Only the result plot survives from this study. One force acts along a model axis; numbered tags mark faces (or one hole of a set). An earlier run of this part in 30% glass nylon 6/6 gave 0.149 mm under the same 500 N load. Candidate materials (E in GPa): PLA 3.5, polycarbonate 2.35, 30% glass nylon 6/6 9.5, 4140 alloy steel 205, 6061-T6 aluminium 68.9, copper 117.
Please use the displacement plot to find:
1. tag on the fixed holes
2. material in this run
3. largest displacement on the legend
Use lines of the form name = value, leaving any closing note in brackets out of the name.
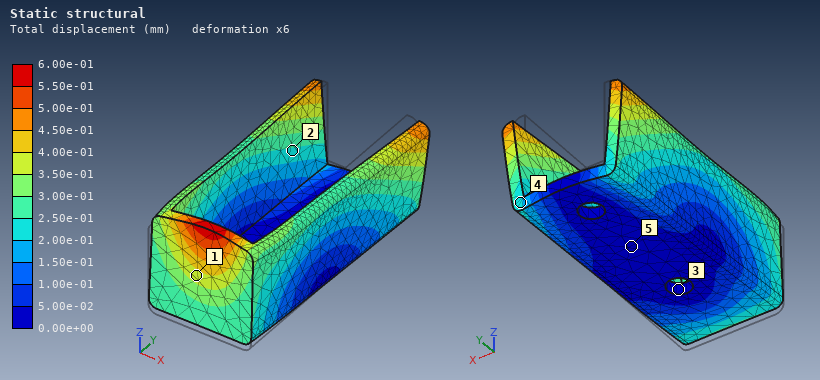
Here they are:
tag on the fixed holes = 3
material in this run = polycarbonate
largest displacement on the legend = 6.00e-01 mm
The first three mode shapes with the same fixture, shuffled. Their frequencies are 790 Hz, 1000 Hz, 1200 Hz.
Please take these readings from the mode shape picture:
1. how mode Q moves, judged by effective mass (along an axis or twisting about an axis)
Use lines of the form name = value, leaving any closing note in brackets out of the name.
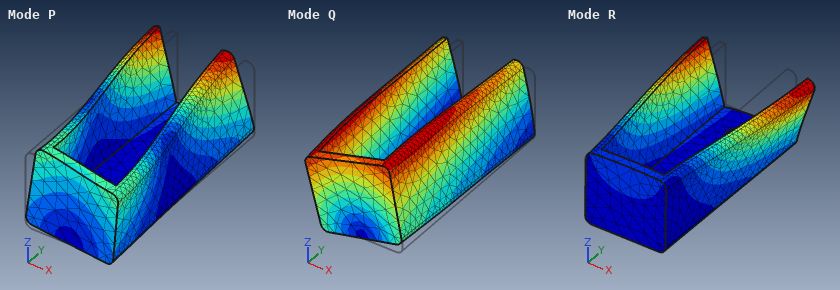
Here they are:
how mode Q moves, judged by effective mass = along X
